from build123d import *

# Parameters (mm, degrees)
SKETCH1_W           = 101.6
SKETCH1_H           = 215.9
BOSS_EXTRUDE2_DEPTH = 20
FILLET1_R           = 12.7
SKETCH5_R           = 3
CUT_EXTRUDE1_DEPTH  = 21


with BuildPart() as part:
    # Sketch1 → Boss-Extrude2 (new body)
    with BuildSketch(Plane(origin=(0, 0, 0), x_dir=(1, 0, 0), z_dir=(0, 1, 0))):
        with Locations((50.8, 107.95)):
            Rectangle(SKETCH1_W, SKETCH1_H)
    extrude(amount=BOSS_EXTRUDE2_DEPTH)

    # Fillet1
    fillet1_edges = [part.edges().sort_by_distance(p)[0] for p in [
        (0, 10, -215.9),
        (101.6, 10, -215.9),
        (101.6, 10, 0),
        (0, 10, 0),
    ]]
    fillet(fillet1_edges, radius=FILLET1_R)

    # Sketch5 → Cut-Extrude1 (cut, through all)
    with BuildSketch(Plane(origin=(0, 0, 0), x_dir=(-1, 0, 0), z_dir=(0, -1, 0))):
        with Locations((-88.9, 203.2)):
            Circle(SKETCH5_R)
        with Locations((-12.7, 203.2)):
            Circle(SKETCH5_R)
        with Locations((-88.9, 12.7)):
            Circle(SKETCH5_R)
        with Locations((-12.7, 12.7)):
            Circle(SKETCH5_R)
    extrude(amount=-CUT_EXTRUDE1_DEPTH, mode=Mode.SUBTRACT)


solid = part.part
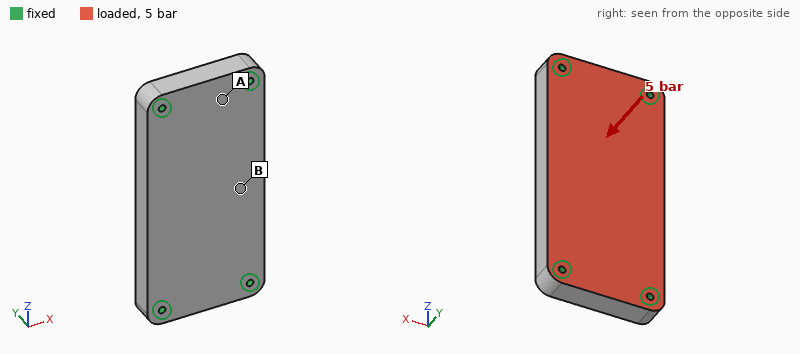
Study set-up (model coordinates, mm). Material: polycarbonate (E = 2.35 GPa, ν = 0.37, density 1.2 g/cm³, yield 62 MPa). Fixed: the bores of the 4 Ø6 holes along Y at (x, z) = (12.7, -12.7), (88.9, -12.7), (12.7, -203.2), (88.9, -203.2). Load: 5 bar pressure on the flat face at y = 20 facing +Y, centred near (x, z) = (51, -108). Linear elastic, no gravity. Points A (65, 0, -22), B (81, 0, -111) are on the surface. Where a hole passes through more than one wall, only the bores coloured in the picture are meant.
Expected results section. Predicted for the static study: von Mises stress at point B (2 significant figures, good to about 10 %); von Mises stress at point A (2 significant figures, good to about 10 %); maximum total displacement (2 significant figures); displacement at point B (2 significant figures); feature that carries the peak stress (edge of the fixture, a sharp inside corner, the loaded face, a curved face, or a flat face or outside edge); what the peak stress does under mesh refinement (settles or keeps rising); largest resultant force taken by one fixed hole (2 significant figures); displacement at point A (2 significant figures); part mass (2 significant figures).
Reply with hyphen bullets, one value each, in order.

- 13 MPa
- 5.8 MPa
- 1.8 mm
- 1.7 mm
- edge of the fixture
- keeps rising
- 2.7 kN
- 0.33 mm
- 520 g
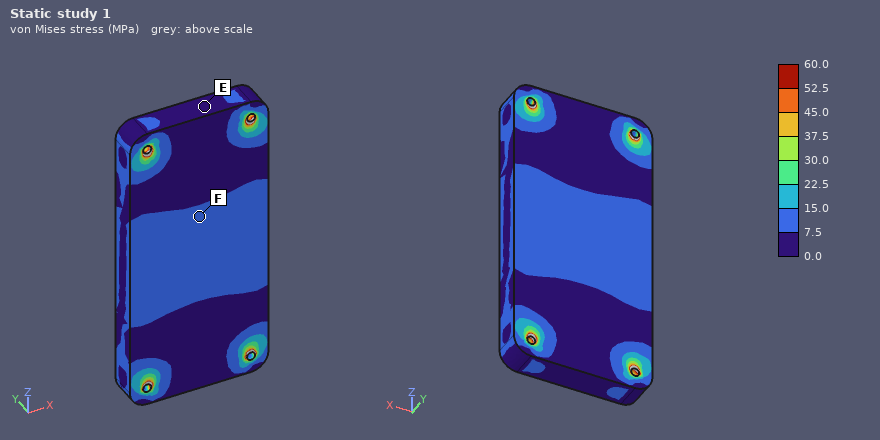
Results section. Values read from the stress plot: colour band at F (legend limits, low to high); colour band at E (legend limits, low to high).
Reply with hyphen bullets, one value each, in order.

- 7.5 to 15.0 MPa
- 0.0 to 7.5 MPa
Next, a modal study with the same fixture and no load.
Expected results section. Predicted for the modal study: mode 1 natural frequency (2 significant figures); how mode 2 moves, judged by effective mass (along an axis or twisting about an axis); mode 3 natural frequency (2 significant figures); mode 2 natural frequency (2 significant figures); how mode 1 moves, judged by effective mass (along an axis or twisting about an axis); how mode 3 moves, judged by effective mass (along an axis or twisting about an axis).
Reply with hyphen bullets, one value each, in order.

- 620 Hz
- twisting about Z
- 1600 Hz
- 1100 Hz
- along Y
- twisting about X
